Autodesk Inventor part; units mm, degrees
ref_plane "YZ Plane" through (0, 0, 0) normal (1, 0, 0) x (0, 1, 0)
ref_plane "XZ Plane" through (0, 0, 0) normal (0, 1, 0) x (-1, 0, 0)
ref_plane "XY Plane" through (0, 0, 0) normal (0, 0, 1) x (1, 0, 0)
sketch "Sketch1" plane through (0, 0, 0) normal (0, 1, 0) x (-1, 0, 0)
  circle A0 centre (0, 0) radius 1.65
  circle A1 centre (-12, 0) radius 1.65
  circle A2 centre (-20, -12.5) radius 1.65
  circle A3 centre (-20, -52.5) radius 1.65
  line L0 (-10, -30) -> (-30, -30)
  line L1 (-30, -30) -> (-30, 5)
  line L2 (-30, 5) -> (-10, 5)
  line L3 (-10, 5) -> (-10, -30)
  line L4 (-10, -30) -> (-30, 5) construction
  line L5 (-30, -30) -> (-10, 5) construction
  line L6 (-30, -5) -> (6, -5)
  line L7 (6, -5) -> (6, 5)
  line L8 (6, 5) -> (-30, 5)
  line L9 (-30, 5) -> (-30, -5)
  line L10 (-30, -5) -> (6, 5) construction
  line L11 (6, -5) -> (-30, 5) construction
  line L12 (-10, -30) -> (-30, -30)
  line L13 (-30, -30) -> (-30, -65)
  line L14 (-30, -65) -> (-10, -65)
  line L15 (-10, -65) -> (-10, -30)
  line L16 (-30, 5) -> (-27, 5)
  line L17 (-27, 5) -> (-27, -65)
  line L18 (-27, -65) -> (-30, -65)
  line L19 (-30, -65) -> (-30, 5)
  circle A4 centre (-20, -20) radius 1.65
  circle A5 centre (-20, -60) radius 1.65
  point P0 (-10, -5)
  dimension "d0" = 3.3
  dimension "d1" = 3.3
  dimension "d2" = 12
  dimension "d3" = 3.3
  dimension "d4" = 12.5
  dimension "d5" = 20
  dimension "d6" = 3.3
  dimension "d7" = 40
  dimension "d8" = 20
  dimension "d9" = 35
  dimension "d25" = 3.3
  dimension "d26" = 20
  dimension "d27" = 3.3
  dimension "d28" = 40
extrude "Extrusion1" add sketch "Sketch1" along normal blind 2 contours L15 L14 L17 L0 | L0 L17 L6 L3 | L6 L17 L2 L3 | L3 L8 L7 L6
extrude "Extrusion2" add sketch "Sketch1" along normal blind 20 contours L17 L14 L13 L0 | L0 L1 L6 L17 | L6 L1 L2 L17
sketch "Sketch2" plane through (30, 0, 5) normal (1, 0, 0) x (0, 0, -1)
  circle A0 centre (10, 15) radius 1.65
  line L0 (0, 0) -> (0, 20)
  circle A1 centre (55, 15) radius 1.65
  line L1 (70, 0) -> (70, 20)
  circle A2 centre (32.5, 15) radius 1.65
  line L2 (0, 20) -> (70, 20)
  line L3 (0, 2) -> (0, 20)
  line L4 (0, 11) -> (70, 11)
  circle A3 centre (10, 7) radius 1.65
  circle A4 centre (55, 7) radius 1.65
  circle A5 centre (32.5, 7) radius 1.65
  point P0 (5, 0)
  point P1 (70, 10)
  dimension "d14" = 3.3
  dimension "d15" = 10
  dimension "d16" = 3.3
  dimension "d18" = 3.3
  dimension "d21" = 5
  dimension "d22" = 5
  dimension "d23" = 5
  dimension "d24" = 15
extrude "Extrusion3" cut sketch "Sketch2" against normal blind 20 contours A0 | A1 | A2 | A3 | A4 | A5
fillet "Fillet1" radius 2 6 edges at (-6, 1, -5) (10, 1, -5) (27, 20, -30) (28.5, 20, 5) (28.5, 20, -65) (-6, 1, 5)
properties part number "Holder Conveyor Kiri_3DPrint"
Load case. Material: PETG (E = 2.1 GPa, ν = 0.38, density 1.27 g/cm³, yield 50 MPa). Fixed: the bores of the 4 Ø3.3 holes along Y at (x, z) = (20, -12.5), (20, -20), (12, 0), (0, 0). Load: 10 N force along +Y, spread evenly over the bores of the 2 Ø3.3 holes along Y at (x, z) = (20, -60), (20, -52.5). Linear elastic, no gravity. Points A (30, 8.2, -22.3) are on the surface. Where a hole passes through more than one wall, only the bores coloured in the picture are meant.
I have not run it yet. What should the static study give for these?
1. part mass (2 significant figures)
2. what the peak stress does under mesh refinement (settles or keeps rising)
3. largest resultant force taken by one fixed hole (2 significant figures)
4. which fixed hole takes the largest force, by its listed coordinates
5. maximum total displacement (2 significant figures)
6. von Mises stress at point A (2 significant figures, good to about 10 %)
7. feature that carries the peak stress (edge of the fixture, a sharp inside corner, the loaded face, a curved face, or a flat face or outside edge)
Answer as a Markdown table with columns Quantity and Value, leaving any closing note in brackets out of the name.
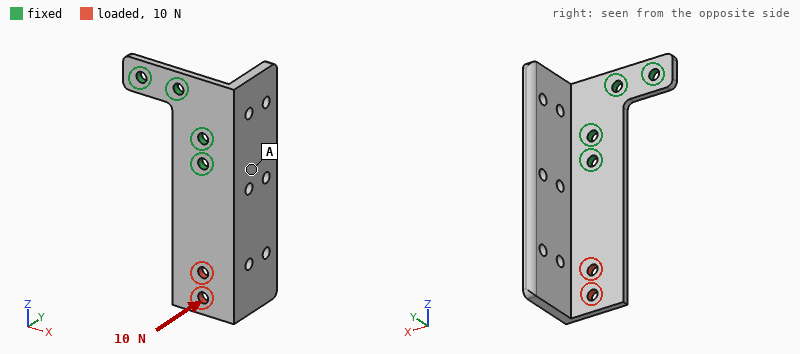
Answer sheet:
| Quantity | Value |
|---|---|
| part mass | 8.4 g |
| what the peak stress does under mesh refinement | keeps rising |
| largest resultant force taken by one fixed hole | 31 N |
| which fixed hole takes the largest force, by its listed coordinates | (20, -20) |
| maximum total displacement | 0.95 mm |
| von Mises stress at point A | 1.1 MPa |
| feature that carries the peak stress | edge of the fixture |
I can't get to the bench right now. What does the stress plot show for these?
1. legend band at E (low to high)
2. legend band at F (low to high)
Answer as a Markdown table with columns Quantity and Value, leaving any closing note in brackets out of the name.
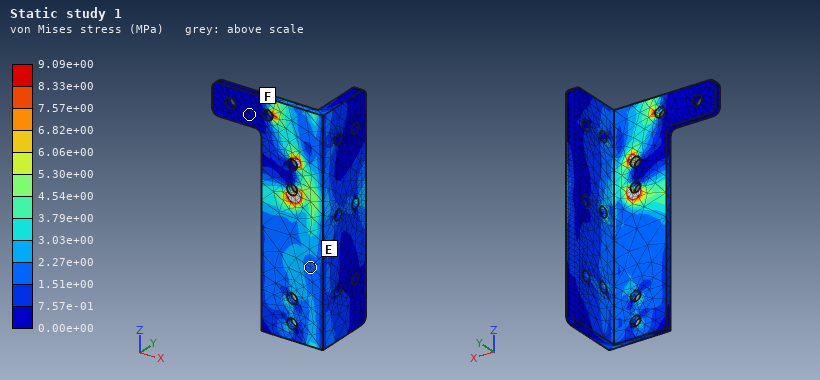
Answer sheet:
| Quantity | Value |
|---|---|
| legend band at E | 1.51e+00 to 2.27e+00 MPa |
| legend band at F | 0.00e+00 to 7.57e-01 MPa |
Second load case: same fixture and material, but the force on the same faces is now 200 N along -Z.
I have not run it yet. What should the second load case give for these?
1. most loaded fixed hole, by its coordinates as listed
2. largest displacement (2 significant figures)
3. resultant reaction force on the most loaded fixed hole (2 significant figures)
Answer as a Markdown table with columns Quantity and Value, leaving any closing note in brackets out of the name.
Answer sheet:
| Quantity | Value |
|---|---|
| most loaded fixed hole, by its coordinates as listed | (20, -20) |
| largest displacement | 0.16 mm |
| resultant reaction force on the most loaded fixed hole | 130 N |
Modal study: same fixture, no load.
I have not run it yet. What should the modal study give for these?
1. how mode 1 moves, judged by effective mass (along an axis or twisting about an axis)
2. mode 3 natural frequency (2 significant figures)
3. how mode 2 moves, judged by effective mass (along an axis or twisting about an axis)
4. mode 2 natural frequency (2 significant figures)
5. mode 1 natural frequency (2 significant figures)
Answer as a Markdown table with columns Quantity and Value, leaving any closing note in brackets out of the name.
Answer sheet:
| Quantity | Value |
|---|---|
| how mode 1 moves, judged by effective mass | along Y |
| mode 3 natural frequency | 920 Hz |
| how mode 2 moves, judged by effective mass | along X |
| mode 2 natural frequency | 460 Hz |
| mode 1 natural frequency | 390 Hz |
